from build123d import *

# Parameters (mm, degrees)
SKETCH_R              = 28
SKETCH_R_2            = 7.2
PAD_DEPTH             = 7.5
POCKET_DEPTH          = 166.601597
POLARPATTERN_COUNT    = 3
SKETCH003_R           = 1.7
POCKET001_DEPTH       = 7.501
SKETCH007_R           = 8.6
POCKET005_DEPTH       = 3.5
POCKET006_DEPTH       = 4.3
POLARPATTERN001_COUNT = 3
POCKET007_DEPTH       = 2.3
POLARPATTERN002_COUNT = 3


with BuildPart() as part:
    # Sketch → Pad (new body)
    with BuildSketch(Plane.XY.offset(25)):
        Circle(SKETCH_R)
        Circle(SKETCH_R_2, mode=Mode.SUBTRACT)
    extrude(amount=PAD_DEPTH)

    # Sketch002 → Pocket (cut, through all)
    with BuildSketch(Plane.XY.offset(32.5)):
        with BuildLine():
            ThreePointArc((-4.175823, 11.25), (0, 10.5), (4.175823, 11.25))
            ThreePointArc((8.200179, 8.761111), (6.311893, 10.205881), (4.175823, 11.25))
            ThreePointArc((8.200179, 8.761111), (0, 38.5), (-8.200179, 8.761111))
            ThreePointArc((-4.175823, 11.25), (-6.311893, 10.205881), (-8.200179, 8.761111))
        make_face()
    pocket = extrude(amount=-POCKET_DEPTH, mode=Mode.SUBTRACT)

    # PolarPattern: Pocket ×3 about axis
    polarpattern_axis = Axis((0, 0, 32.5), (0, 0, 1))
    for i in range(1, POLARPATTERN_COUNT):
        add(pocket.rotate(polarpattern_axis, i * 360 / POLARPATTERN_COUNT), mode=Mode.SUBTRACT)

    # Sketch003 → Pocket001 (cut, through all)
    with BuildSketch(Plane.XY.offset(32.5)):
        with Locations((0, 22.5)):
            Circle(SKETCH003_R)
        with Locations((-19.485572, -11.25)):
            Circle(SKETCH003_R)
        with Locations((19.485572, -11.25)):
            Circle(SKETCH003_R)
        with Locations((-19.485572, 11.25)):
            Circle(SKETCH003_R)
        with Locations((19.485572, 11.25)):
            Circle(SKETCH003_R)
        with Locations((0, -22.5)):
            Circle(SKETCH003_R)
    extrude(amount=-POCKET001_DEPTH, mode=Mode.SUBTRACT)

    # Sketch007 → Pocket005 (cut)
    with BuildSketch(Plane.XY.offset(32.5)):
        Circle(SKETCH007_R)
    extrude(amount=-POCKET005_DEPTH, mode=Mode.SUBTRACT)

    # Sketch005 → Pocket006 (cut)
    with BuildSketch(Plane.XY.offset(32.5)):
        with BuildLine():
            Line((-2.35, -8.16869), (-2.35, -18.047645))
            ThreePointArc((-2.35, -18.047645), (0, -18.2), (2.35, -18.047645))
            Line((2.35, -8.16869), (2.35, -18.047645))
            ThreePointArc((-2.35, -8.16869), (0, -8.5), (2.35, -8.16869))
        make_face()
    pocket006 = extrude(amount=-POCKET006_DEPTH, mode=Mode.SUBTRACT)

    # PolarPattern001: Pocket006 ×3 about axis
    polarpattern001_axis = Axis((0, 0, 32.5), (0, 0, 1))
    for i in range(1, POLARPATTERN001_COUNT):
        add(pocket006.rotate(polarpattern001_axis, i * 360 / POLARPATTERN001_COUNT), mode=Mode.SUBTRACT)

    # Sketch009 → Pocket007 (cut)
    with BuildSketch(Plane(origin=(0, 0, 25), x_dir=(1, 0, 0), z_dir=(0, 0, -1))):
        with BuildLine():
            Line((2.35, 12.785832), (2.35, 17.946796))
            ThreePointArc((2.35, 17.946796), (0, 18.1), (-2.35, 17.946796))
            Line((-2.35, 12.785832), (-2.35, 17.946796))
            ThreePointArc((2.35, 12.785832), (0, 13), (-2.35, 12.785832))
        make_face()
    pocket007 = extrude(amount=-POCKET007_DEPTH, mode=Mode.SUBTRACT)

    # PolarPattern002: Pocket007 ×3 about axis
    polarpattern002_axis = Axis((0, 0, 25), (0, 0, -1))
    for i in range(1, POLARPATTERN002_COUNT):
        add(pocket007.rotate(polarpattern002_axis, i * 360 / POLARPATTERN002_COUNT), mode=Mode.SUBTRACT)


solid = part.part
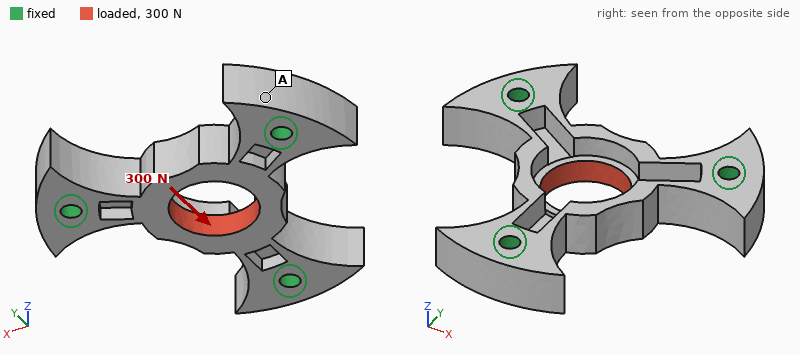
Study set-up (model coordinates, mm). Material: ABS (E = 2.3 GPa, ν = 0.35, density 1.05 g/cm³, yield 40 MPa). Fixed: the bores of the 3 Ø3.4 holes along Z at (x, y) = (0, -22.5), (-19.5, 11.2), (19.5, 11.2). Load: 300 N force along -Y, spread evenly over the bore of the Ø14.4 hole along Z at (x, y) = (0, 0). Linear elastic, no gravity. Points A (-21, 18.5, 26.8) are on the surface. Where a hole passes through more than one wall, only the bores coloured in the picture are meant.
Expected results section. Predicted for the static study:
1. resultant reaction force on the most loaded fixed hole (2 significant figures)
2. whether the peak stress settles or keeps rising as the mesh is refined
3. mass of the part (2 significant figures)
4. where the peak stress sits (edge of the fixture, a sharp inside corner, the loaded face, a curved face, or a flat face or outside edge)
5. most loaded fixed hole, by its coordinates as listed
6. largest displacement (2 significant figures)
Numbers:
140 N
keeps rising
5.7 g
a sharp inside corner
(0, -22.5)
0.16 mm
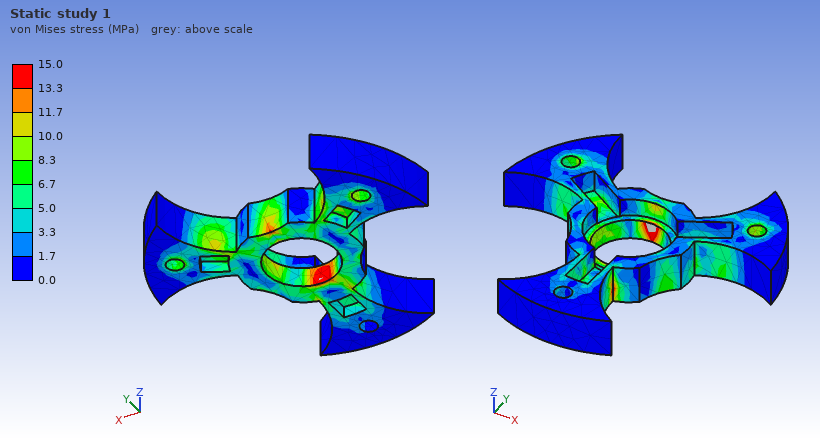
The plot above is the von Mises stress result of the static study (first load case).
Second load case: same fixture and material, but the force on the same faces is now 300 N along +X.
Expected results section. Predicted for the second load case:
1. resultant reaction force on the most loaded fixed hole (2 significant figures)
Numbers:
130 N
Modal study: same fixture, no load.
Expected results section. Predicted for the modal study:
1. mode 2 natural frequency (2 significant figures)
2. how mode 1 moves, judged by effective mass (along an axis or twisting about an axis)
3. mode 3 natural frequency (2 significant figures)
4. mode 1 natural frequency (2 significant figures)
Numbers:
5900 Hz
along Z
5900 Hz
5500 Hz
